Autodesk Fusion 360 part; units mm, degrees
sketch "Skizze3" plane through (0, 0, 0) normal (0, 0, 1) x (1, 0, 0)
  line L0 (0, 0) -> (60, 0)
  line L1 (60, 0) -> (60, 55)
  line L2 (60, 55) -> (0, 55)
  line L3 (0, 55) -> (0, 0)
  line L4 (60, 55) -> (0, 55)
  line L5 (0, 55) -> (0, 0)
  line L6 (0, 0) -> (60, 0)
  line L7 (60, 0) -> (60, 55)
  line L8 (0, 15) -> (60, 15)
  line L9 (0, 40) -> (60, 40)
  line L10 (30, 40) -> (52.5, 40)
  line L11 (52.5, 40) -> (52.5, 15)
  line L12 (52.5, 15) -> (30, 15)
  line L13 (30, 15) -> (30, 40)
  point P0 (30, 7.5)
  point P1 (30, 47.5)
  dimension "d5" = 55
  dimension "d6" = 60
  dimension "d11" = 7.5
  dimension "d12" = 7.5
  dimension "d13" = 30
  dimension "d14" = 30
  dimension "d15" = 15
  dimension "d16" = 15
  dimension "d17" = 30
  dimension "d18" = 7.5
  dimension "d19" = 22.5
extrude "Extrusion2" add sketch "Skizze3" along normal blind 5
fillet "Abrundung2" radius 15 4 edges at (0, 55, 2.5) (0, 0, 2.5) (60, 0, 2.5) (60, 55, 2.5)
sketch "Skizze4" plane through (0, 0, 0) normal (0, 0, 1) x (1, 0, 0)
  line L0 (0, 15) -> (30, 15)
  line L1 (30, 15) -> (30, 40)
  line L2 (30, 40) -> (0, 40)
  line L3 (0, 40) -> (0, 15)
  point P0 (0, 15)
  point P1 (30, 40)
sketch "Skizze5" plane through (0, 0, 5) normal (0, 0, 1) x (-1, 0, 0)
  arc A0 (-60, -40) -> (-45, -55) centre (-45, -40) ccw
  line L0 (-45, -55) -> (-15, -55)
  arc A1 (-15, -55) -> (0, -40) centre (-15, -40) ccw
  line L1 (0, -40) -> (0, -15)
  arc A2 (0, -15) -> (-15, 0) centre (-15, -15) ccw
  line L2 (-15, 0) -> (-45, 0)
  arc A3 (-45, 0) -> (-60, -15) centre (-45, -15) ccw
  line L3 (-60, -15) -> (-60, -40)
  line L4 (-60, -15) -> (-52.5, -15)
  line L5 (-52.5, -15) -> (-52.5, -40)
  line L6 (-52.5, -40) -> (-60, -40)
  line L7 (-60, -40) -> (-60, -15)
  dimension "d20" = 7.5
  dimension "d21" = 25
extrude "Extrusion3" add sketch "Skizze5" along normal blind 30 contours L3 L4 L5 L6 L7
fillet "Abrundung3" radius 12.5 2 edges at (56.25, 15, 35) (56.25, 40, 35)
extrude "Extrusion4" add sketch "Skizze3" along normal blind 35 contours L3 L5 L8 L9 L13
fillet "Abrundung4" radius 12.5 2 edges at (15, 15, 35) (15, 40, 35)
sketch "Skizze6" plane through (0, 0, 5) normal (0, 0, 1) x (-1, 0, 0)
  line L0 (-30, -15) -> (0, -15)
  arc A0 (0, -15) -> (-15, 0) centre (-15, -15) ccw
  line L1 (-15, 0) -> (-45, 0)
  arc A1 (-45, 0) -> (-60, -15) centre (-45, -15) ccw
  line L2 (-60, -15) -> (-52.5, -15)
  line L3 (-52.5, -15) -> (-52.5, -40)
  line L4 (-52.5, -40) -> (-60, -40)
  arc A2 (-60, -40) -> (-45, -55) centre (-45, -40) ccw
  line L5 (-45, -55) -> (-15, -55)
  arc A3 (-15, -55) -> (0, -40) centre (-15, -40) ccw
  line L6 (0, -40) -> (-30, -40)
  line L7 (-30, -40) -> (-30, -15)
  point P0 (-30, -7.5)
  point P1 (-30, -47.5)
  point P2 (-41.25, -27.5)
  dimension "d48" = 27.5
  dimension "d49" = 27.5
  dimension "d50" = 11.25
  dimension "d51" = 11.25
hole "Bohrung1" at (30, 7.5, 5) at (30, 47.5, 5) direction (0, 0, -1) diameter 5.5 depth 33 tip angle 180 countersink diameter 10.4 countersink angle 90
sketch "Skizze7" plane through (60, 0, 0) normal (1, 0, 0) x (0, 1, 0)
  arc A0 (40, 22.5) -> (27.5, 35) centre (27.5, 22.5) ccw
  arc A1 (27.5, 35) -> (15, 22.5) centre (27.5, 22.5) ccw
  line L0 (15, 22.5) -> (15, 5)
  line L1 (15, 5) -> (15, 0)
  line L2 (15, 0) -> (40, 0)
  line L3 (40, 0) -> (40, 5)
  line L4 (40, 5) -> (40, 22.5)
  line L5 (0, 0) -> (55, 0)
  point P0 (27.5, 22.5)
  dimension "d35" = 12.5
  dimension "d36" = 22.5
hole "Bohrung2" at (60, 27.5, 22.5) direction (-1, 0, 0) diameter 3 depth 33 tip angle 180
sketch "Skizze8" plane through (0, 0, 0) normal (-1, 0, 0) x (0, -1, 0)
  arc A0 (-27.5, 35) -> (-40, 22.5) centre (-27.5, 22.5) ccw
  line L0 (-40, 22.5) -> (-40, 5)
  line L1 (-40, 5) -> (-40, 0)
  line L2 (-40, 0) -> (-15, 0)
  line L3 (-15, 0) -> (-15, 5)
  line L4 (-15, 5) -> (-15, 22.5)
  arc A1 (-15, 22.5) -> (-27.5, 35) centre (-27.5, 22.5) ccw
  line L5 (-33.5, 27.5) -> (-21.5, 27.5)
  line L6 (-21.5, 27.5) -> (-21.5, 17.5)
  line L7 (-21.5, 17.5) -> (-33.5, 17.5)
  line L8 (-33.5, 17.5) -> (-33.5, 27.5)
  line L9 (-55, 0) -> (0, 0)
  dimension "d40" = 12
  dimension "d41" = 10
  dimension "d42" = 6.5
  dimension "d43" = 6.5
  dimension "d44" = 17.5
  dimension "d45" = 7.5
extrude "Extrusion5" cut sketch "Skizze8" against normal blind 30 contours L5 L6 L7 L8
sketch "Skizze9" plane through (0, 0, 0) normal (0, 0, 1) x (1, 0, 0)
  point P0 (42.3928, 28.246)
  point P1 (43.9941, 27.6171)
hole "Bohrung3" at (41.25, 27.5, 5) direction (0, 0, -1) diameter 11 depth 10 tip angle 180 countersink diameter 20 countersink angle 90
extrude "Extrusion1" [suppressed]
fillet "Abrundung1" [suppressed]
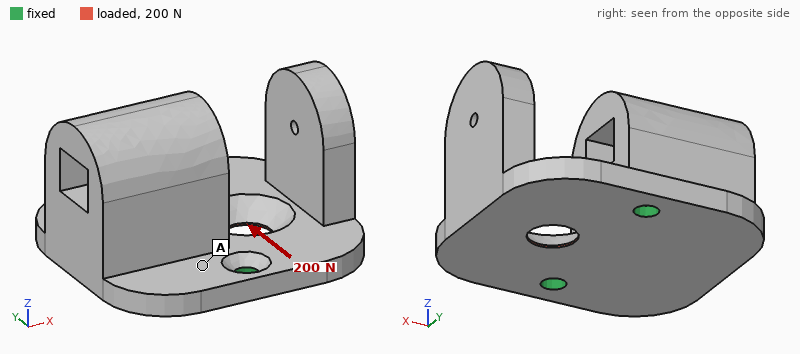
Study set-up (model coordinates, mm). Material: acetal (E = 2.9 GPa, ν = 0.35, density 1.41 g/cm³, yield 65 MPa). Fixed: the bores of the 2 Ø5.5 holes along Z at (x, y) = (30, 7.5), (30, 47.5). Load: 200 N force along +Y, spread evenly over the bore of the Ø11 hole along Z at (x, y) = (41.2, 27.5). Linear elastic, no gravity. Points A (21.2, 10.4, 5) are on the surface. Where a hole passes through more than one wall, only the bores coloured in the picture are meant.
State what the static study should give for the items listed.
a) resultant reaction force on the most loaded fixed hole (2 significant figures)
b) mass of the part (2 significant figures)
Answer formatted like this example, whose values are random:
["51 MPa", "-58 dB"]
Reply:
["110 N", "51 g"]
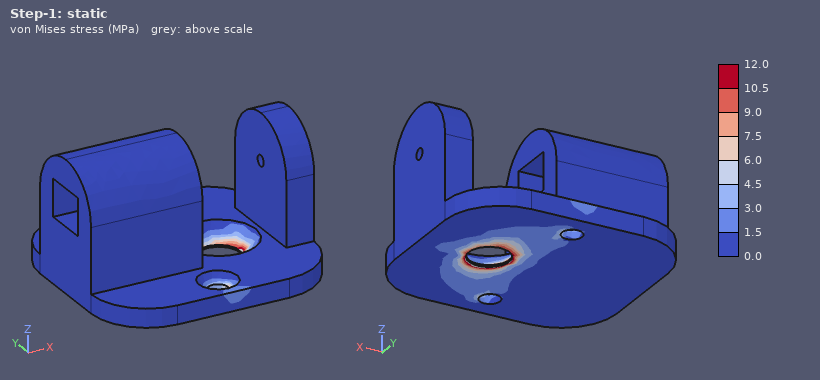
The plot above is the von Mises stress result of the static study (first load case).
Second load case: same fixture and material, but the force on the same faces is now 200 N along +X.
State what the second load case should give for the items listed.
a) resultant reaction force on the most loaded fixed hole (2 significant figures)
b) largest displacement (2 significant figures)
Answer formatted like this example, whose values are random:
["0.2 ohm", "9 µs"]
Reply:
["100 N", "0.16 mm"]
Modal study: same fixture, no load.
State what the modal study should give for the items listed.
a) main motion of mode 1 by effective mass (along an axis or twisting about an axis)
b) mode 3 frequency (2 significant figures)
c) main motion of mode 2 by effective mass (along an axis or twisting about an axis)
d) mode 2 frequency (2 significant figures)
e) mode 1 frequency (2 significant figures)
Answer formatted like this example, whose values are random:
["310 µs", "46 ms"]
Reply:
["along X", "1000 Hz", "along Z", "560 Hz", "390 Hz"]
